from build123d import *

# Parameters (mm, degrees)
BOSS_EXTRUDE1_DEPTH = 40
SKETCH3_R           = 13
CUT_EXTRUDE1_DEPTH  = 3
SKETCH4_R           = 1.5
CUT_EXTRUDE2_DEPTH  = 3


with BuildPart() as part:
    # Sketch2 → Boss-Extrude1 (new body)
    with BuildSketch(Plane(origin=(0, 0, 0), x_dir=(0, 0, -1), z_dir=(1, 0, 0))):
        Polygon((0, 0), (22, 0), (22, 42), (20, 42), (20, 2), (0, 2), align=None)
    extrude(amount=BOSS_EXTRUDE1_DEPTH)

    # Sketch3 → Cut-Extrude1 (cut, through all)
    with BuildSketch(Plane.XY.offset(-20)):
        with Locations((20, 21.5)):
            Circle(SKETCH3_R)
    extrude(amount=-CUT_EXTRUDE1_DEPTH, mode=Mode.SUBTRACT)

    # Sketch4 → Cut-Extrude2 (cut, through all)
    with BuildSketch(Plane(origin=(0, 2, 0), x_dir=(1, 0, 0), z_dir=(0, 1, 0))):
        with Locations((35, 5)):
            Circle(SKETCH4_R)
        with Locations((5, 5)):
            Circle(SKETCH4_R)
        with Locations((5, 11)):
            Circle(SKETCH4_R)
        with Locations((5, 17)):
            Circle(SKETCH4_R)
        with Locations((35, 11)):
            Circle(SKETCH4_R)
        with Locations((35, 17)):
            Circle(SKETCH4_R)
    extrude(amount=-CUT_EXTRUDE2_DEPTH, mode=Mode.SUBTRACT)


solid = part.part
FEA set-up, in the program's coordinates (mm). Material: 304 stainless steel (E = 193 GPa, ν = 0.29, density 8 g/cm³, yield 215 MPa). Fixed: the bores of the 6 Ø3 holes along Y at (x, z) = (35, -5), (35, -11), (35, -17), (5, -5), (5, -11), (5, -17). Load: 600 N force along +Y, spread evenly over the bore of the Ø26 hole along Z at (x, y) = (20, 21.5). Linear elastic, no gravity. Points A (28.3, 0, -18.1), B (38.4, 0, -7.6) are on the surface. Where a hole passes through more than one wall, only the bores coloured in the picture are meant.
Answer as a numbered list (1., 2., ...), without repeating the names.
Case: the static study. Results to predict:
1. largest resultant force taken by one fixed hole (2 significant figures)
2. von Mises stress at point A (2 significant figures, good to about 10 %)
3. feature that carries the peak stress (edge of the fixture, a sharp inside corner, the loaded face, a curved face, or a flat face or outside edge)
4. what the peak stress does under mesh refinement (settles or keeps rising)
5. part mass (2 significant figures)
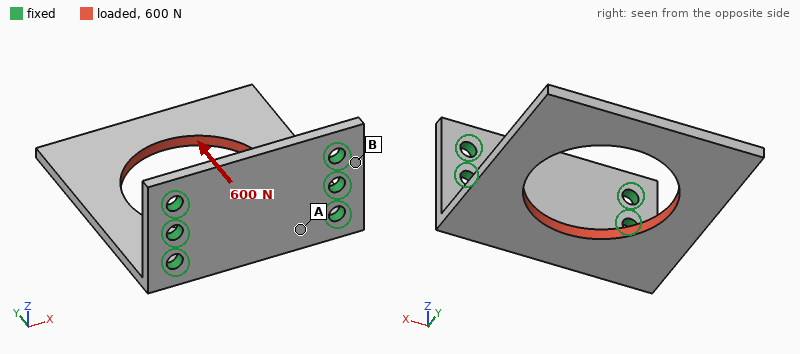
1. 330 N
2. 20 MPa
3. edge of the fixture
4. keeps rising
5. 31 g
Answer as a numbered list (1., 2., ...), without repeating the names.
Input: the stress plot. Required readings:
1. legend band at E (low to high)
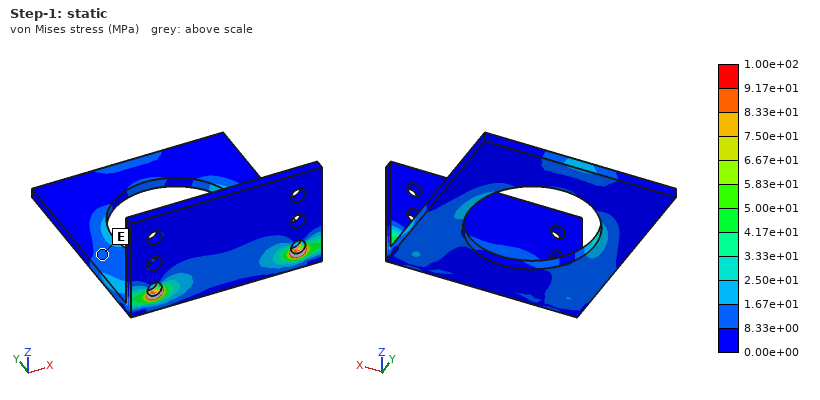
1. 8.33e+00 to 1.67e+01 MPa
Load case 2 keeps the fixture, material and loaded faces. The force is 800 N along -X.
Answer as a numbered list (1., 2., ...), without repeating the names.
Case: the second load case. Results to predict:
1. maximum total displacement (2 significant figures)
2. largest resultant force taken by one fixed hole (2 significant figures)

1. 53 µm
2. 630 N
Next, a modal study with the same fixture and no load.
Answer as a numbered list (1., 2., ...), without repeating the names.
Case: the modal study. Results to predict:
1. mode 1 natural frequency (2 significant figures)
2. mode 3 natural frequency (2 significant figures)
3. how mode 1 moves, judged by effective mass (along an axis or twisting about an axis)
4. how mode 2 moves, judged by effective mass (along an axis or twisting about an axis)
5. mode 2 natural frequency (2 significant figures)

1. 740 Hz
2. 4800 Hz
3. along Z
4. twisting about Y
5. 1800 Hz
